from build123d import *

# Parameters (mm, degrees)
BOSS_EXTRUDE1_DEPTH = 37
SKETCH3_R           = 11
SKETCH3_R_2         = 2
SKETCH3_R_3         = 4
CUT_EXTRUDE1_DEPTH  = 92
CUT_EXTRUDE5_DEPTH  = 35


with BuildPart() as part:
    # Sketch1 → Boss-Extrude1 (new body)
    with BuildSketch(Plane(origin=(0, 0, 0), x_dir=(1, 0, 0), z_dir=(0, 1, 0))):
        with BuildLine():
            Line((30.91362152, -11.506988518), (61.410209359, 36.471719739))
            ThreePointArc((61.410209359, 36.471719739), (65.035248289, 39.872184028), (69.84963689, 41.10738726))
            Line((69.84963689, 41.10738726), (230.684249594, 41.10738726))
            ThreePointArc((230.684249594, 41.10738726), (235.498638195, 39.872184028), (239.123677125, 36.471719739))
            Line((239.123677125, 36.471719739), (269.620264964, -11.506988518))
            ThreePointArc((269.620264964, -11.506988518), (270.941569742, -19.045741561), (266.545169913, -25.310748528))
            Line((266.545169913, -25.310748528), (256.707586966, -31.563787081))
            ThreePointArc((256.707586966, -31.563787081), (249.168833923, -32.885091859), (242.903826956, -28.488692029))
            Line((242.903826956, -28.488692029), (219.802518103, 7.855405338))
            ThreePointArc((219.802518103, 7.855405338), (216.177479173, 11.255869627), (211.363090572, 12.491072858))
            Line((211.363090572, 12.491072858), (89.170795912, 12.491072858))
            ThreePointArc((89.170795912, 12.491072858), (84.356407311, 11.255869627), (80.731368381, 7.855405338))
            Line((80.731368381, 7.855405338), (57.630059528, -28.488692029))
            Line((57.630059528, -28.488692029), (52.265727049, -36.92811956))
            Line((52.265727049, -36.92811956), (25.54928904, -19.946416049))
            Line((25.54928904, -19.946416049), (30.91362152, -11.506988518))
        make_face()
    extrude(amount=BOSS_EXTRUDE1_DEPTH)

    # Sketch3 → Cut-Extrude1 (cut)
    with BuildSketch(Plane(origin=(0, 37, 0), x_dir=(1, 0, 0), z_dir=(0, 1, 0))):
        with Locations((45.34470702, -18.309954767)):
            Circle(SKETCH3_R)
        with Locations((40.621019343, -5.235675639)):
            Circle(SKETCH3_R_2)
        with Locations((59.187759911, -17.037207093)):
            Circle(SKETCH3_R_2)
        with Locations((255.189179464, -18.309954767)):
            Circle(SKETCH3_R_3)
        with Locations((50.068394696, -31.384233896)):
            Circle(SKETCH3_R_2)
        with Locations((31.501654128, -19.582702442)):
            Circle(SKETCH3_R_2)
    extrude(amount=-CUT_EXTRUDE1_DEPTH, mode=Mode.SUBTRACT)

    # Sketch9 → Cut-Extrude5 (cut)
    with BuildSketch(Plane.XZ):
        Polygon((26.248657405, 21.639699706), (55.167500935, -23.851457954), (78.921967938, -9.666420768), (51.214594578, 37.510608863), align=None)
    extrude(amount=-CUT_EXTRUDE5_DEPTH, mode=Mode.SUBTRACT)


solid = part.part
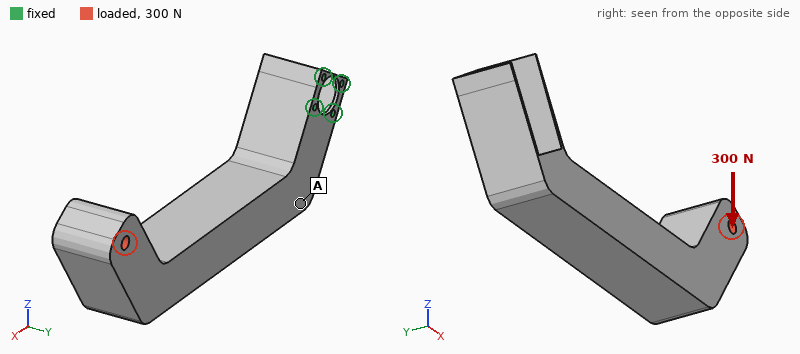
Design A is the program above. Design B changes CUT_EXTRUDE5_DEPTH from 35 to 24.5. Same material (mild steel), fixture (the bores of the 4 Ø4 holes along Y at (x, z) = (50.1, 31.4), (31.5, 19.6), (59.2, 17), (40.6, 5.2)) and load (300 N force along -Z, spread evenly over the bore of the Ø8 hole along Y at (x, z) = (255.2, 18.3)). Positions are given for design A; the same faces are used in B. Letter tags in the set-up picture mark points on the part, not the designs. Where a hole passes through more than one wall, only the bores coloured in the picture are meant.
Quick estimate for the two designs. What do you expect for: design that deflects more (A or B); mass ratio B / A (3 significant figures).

A
1.04
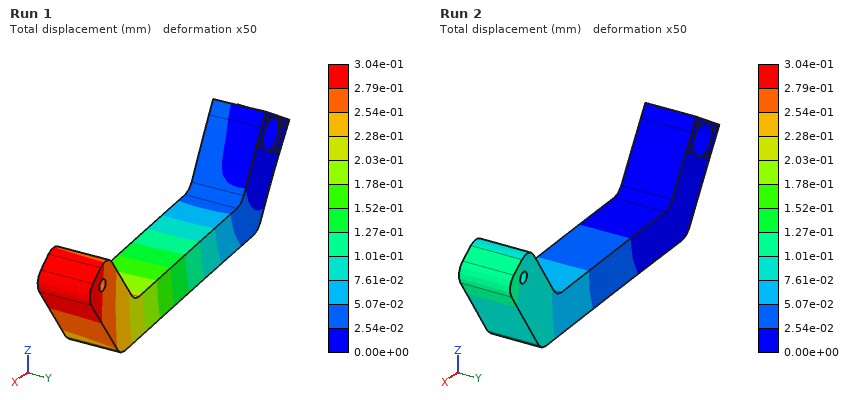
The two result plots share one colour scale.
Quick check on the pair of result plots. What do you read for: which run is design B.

Run 2
